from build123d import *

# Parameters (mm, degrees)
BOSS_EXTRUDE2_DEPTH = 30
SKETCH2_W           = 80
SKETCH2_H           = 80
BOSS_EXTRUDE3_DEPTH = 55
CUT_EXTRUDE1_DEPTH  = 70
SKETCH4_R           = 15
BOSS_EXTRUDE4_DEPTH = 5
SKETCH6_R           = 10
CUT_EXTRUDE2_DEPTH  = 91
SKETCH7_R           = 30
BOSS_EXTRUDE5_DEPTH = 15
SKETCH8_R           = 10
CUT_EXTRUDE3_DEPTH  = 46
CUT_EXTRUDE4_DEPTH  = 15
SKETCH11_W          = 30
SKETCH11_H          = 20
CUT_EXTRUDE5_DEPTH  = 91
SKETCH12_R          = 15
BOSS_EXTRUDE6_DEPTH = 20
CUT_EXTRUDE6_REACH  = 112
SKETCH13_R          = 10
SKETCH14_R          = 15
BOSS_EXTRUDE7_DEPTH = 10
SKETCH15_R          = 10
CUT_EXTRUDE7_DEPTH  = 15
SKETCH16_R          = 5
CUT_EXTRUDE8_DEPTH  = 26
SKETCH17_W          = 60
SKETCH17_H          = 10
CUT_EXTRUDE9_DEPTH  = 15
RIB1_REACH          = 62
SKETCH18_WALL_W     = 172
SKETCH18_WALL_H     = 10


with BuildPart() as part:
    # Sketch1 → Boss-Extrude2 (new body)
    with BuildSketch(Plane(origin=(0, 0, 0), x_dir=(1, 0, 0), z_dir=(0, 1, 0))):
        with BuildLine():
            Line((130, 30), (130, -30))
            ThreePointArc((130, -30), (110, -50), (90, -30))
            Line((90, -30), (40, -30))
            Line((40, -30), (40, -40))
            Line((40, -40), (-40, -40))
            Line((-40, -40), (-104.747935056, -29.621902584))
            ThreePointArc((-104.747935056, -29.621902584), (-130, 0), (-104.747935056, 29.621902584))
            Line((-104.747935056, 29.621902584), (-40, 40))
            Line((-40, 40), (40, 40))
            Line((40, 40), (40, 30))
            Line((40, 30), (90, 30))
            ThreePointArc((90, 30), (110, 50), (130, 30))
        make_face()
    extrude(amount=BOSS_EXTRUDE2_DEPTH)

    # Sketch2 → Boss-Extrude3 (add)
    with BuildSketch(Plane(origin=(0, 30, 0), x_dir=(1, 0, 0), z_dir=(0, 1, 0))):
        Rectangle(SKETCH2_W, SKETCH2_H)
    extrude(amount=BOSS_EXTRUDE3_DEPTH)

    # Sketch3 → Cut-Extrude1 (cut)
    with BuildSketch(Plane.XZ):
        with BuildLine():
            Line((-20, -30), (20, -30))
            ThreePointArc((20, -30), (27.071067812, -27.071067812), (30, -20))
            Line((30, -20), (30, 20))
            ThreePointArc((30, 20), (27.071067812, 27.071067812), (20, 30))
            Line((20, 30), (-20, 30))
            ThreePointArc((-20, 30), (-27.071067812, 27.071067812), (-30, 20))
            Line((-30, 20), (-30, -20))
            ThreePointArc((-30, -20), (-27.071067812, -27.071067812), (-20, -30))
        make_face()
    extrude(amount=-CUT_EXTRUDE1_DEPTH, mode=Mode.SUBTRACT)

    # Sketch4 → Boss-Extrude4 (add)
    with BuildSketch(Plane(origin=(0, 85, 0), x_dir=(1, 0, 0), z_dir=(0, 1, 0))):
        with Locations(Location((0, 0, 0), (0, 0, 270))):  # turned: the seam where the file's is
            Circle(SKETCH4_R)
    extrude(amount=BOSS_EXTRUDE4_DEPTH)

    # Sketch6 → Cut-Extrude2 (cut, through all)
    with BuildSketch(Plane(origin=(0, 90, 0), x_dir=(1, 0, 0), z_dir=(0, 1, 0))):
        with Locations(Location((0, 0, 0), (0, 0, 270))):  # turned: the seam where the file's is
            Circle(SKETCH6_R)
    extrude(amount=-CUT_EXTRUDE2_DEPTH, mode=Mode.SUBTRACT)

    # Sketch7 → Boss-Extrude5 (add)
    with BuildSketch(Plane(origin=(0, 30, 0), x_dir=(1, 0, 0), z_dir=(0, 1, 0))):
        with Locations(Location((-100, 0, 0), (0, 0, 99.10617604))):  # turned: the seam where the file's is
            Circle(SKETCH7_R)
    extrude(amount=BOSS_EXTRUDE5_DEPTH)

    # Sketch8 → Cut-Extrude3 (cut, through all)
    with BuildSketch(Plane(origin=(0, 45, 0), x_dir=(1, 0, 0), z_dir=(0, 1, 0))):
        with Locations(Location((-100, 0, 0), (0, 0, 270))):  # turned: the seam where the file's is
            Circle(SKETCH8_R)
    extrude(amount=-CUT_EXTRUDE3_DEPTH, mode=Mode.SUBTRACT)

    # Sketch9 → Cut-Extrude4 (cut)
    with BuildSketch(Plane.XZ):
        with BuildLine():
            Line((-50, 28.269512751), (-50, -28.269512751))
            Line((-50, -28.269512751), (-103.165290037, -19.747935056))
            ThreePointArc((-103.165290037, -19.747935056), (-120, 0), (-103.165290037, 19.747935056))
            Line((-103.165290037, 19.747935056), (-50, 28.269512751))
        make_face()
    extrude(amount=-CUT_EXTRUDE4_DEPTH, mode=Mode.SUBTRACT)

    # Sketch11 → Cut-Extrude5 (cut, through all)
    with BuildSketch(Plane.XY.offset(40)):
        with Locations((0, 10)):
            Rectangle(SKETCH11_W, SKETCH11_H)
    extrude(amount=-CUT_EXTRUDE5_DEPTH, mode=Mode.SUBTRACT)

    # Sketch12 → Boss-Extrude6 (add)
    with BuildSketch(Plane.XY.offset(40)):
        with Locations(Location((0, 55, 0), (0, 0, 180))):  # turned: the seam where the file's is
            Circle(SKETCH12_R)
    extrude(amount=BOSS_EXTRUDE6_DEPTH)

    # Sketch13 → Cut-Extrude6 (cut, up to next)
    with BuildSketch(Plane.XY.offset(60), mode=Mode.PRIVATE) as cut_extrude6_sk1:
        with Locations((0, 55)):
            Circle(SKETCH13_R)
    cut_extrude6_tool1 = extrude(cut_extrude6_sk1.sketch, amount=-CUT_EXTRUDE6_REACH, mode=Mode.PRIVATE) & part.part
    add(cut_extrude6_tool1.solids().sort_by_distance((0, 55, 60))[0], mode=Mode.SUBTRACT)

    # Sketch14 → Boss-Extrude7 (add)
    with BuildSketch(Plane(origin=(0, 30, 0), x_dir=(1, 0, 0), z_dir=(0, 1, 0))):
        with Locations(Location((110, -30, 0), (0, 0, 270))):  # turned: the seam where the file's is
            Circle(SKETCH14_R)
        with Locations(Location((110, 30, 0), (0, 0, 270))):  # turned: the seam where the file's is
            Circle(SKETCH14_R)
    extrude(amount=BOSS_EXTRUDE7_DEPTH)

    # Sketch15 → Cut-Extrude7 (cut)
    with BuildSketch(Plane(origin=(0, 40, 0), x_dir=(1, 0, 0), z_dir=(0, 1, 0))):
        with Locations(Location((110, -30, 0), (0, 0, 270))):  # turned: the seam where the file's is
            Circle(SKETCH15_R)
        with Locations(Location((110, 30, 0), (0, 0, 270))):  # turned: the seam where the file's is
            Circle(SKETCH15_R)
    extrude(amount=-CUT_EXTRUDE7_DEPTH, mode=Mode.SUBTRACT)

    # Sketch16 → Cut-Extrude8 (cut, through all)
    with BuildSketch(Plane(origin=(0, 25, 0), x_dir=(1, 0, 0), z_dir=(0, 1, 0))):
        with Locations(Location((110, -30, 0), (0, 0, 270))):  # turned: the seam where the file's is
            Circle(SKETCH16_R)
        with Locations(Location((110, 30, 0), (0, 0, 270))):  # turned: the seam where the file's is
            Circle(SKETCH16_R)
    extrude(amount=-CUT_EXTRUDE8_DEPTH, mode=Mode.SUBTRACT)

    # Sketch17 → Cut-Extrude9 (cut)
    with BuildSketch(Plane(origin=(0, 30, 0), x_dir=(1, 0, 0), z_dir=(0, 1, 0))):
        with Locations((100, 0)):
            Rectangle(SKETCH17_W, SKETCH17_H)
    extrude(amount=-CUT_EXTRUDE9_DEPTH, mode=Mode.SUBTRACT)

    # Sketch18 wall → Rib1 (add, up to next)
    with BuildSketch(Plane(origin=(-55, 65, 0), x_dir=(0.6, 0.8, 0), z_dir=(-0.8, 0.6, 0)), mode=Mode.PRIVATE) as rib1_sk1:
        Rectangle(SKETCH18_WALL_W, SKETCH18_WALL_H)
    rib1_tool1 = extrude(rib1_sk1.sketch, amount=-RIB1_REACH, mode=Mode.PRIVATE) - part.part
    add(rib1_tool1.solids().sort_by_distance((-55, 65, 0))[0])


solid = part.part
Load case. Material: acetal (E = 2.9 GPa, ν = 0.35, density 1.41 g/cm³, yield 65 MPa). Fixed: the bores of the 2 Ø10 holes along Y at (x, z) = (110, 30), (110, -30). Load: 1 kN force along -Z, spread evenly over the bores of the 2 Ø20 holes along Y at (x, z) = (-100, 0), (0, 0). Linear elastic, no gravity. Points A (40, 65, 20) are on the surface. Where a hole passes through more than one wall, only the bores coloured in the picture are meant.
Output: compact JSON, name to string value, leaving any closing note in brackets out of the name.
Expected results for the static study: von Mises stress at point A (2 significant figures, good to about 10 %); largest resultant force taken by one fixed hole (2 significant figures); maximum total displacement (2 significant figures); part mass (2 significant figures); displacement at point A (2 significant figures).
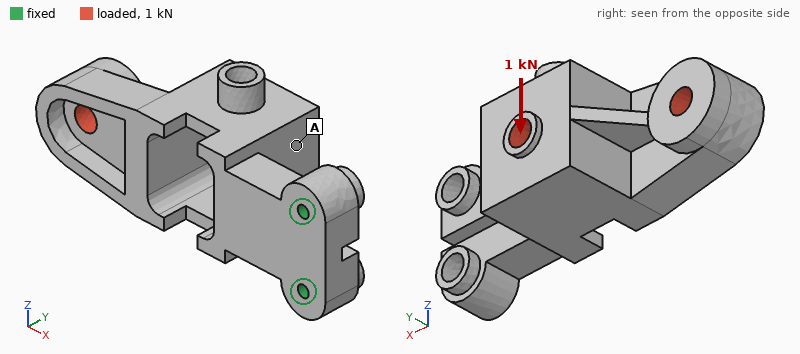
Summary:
{"von Mises stress at point A": "2.3 MPa", "largest resultant force taken by one fixed hole": "2.9 kN", "maximum total displacement": "3.0 mm", "part mass": "910 g", "displacement at point A": "0.53 mm"}
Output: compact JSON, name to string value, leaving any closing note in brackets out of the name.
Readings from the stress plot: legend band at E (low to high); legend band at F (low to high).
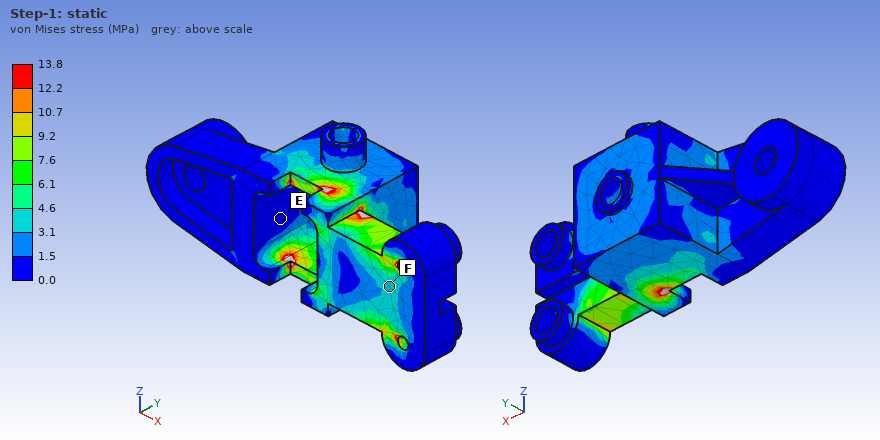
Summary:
{"legend band at E": "0.0 to 1.5 MPa", "legend band at F": "3.1 to 4.6 MPa"}
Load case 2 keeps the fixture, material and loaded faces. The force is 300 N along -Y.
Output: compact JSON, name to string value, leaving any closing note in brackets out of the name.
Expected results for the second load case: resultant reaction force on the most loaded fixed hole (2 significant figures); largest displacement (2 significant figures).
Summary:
{"resultant reaction force on the most loaded fixed hole": "190 N", "largest displacement": "2.9 mm"}
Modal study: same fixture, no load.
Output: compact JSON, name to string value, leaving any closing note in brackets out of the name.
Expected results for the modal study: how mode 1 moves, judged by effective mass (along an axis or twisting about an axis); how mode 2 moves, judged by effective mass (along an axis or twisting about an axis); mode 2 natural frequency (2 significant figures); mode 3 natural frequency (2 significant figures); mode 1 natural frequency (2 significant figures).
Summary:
{"how mode 1 moves, judged by effective mass": "along Y", "how mode 2 moves, judged by effective mass": "along Z", "mode 2 natural frequency": "160 Hz", "mode 3 natural frequency": "320 Hz", "mode 1 natural frequency": "92 Hz"}
